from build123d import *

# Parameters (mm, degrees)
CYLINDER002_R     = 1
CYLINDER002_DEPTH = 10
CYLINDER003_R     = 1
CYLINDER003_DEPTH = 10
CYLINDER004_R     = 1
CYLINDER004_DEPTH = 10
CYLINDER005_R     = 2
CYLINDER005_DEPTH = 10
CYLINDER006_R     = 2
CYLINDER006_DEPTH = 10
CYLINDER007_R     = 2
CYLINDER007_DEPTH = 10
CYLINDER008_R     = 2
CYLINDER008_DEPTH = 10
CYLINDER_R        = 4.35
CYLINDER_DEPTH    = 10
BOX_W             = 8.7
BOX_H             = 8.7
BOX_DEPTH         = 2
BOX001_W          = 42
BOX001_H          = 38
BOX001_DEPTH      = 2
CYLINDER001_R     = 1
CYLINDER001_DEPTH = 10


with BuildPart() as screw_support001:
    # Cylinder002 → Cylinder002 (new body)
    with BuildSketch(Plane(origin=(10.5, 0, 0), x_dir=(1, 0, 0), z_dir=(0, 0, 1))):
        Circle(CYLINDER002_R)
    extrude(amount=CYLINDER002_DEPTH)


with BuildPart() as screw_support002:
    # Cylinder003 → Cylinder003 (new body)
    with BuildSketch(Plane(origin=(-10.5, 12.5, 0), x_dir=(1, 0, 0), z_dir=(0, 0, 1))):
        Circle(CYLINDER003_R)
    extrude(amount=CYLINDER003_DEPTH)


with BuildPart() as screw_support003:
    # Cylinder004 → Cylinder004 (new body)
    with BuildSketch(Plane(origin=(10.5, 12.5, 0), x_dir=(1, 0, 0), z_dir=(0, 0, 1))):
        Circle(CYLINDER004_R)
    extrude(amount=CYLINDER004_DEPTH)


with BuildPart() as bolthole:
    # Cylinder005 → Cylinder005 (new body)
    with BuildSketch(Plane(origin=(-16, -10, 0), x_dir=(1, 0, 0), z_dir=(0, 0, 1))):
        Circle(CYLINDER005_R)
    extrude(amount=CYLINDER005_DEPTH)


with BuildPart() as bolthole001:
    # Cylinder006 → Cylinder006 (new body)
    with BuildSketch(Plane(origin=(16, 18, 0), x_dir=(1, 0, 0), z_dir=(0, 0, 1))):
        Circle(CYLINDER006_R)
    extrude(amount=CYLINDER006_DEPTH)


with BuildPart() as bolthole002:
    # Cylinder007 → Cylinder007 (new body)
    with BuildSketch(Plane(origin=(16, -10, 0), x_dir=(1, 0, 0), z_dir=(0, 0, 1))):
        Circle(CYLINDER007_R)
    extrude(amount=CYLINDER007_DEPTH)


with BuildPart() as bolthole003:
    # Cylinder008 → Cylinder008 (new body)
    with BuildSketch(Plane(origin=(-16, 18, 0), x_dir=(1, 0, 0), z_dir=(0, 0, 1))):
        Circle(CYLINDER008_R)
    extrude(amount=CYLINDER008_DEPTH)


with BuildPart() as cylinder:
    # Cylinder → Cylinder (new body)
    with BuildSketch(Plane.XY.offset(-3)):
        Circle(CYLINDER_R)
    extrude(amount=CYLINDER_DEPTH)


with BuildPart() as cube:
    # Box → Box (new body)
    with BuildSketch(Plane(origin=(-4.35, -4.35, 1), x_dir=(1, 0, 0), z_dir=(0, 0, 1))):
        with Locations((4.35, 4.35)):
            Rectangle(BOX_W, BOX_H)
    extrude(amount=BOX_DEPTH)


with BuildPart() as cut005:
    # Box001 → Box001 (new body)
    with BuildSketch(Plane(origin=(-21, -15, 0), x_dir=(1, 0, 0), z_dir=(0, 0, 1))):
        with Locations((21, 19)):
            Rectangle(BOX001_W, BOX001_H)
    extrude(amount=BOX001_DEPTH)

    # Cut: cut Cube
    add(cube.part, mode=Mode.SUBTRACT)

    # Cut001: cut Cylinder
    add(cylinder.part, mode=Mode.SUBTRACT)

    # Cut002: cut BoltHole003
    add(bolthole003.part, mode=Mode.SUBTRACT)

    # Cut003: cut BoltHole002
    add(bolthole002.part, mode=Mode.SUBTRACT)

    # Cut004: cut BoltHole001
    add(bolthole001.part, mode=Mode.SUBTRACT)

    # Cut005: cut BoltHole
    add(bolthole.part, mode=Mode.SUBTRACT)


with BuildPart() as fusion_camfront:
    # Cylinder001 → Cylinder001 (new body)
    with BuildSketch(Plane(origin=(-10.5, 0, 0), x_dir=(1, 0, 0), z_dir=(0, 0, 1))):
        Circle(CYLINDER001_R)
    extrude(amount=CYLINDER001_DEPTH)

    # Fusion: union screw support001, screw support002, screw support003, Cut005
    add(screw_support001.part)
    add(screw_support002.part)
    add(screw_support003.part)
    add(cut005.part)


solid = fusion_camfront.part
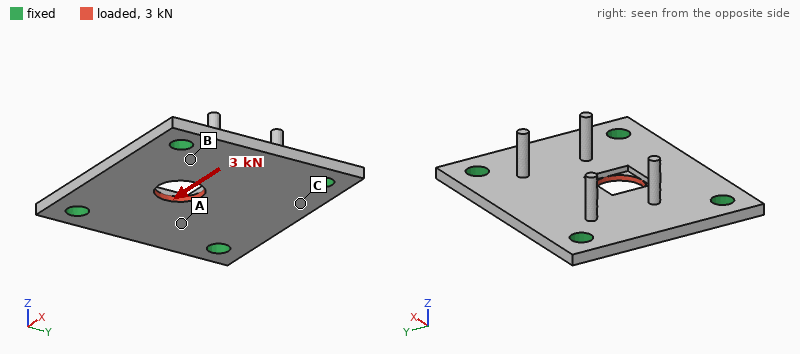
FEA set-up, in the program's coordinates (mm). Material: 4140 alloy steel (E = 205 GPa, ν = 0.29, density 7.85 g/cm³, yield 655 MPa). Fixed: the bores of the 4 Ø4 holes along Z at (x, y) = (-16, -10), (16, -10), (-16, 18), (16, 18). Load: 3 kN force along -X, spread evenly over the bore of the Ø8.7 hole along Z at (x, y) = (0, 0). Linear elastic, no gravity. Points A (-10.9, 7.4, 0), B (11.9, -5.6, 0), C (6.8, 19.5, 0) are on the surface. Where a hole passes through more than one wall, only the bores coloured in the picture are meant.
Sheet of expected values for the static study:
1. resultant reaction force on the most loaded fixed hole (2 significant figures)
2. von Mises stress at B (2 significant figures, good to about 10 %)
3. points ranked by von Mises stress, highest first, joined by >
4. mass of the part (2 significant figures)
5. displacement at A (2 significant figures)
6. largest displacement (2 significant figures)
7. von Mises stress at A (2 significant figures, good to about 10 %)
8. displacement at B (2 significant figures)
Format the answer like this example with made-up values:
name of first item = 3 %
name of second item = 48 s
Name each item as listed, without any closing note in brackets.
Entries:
resultant reaction force on the most loaded fixed hole = 950 N
von Mises stress at B = 51 MPa
points ranked by von Mises stress, highest first, joined by > = B > A > C
mass of the part = 24 g
displacement at A = 2.8 µm
largest displacement = 5.5 µm
von Mises stress at A = 32 MPa
displacement at B = 1.6 µm
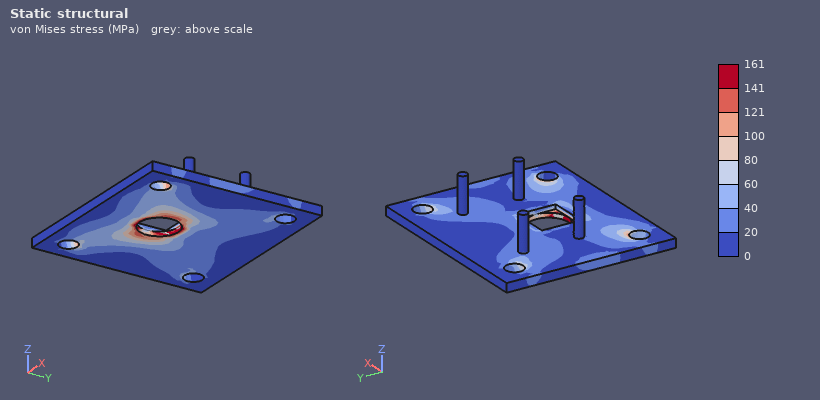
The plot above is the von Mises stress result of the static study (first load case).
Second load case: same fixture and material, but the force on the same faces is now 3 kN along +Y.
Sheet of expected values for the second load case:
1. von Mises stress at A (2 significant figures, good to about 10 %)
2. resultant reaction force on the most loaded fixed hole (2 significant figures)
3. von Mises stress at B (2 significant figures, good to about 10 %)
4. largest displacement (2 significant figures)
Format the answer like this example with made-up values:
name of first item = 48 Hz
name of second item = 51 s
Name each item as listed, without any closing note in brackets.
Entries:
von Mises stress at A = 45 MPa
resultant reaction force on the most loaded fixed hole = 870 N
von Mises stress at B = 55 MPa
largest displacement = 7.7 µm
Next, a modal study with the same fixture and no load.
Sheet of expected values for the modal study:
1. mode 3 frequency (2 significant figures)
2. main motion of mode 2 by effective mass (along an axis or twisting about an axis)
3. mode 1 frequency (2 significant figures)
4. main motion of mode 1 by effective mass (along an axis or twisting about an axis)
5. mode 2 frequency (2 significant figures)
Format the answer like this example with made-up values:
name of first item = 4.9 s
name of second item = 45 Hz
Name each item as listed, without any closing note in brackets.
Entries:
mode 3 frequency = 14 kHz
main motion of mode 2 by effective mass = twisting about X
mode 1 frequency = 8900 Hz
main motion of mode 1 by effective mass = along Z
mode 2 frequency = 13 kHz
